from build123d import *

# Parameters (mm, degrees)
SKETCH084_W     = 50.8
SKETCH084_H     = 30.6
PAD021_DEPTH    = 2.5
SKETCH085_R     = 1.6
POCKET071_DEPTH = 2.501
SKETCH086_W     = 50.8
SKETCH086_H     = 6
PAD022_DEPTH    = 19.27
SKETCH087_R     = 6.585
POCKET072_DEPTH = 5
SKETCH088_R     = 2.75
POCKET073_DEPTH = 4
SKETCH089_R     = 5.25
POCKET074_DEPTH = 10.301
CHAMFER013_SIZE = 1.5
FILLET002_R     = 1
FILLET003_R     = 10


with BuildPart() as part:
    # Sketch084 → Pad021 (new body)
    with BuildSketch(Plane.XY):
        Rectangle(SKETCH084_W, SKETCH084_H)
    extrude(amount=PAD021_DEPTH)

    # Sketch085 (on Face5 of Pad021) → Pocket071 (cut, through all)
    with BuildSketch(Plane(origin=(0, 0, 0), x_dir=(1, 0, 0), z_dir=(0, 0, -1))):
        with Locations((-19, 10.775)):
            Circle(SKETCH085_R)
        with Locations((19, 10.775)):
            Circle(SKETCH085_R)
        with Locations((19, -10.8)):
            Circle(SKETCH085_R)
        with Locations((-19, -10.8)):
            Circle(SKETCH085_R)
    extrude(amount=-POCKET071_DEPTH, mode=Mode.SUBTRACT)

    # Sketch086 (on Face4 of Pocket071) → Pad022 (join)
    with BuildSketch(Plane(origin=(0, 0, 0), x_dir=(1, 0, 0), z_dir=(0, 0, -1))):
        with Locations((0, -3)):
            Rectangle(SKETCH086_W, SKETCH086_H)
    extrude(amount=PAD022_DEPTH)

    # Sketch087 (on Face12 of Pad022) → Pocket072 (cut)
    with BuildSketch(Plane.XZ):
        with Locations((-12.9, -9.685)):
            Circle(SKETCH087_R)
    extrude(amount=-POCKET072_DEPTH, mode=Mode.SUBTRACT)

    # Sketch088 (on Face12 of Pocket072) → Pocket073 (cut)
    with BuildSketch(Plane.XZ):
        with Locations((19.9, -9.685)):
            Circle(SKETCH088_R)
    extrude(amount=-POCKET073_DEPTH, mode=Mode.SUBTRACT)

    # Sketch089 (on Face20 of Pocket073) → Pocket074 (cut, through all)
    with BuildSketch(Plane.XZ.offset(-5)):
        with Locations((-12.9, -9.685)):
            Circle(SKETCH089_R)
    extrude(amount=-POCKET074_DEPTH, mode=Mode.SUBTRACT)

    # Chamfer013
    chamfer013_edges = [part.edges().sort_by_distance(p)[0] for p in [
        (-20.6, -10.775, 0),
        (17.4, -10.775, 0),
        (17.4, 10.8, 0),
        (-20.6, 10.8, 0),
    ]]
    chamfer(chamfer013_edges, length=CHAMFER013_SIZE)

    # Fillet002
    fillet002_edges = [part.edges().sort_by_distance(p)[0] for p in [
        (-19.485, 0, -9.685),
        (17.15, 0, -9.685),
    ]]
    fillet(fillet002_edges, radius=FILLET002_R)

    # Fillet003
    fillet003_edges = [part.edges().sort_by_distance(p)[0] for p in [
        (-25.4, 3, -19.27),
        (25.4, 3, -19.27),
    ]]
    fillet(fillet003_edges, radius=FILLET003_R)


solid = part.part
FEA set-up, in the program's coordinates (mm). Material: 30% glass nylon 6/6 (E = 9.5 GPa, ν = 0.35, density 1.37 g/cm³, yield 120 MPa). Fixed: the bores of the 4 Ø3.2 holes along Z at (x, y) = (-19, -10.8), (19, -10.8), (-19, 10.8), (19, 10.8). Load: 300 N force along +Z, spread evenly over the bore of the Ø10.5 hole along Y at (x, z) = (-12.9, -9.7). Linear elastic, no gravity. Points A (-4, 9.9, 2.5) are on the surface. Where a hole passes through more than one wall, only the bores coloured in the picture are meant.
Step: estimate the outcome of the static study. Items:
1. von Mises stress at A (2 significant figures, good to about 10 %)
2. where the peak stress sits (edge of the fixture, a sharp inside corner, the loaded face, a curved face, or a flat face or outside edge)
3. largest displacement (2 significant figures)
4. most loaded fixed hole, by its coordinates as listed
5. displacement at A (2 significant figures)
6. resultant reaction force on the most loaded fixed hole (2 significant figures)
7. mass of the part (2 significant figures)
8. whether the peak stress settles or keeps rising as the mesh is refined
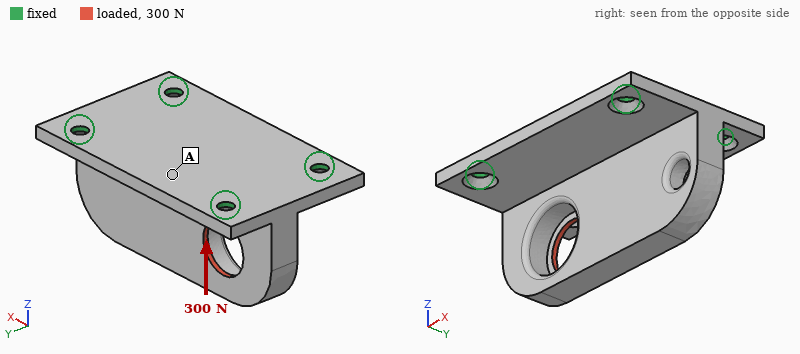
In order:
4.9 MPa
edge of the fixture
68 µm
(-19, 10.8)
39 µm
230 N
12 g
keeps rising
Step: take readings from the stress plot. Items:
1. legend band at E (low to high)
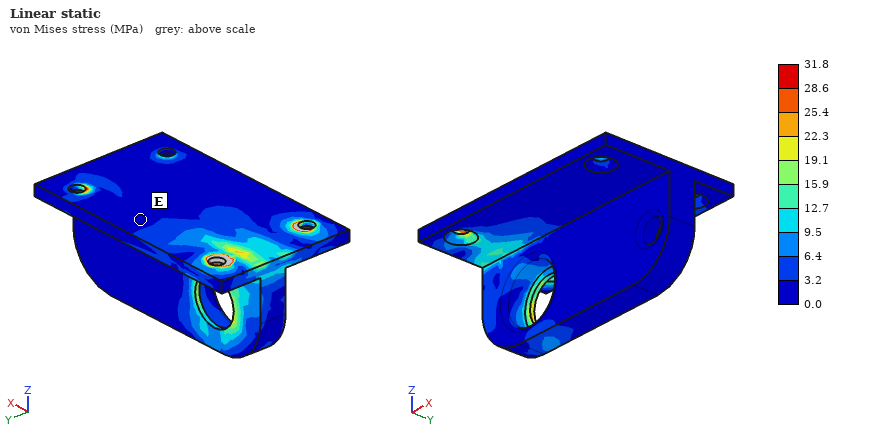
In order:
0.0 to 3.2 MPa
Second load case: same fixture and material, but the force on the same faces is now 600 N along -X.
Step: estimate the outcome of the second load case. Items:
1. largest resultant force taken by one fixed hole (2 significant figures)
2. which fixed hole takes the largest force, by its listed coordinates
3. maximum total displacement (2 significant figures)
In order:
280 N
(-19, 10.8)
0.11 mm
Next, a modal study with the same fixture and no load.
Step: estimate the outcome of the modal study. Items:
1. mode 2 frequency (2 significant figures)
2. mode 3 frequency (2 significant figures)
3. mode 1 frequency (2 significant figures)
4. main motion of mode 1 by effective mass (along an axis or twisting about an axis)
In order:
5000 Hz
5100 Hz
2800 Hz
along Y
